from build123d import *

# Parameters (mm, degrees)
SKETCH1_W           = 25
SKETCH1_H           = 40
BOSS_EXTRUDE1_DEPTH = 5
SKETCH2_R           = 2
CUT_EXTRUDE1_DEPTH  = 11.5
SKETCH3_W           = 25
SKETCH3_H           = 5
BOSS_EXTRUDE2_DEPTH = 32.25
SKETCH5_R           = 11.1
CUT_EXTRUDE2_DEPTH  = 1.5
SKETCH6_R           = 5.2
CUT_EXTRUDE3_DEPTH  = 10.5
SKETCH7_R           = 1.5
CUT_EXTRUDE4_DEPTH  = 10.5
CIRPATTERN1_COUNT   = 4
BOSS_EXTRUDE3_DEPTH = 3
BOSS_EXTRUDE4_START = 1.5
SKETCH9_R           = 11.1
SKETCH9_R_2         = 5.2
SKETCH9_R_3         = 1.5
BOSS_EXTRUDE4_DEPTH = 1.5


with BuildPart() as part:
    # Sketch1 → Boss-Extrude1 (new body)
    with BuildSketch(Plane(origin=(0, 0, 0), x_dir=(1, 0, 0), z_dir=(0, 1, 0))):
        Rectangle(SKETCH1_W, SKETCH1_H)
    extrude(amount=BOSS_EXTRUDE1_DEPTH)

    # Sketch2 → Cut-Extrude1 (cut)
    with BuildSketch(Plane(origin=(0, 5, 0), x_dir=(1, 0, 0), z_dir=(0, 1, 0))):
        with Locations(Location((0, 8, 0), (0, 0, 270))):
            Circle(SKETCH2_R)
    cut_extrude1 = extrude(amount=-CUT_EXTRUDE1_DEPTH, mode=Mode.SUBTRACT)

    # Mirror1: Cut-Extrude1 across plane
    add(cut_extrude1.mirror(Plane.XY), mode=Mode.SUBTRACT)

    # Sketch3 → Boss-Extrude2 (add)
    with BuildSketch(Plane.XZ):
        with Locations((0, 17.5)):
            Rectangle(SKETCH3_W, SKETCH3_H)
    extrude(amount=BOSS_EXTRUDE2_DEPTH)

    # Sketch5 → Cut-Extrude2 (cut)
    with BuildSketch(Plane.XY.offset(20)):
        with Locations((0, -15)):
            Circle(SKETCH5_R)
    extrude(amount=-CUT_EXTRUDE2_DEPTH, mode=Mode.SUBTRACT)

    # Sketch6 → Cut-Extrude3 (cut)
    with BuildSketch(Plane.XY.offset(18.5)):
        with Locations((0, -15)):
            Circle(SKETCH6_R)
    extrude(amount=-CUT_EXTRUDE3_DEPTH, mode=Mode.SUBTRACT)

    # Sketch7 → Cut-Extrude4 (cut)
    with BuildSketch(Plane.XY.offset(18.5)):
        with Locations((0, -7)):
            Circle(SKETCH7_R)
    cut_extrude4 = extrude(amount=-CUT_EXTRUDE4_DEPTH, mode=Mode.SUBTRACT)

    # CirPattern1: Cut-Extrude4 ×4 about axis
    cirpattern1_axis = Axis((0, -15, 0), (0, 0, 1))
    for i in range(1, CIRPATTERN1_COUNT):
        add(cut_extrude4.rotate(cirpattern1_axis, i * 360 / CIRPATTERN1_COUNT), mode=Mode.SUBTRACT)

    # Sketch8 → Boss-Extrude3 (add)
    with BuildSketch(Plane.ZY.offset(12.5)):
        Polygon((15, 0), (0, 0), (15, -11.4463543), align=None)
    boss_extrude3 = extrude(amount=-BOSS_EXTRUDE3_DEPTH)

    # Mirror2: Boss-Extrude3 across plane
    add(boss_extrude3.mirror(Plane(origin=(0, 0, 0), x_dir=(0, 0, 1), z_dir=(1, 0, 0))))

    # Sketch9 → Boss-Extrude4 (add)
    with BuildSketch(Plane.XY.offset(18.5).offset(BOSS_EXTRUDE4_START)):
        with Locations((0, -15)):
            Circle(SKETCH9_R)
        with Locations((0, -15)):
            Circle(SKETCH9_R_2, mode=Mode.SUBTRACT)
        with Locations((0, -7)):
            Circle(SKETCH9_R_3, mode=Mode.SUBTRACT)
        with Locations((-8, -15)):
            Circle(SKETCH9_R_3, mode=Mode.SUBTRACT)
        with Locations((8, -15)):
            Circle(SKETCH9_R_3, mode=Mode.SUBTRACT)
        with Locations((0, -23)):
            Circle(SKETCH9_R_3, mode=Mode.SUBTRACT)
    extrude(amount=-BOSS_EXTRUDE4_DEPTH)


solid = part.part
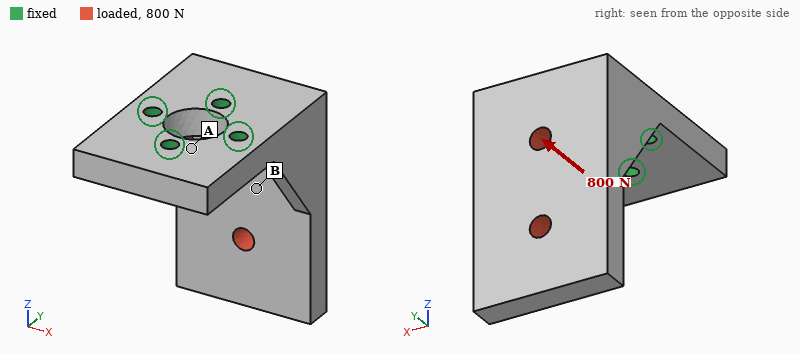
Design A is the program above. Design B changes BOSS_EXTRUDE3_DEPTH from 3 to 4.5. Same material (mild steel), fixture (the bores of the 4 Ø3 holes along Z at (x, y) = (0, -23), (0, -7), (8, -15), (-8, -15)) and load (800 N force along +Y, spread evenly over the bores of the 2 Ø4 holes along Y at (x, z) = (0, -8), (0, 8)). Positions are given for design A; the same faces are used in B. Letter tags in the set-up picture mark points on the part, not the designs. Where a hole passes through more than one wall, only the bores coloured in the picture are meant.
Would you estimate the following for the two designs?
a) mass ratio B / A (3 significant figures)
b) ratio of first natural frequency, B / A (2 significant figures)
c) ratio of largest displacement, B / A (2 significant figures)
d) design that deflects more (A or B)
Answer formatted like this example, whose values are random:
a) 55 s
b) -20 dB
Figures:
a) 1.03
b) 1.1
c) 0.85
d) A
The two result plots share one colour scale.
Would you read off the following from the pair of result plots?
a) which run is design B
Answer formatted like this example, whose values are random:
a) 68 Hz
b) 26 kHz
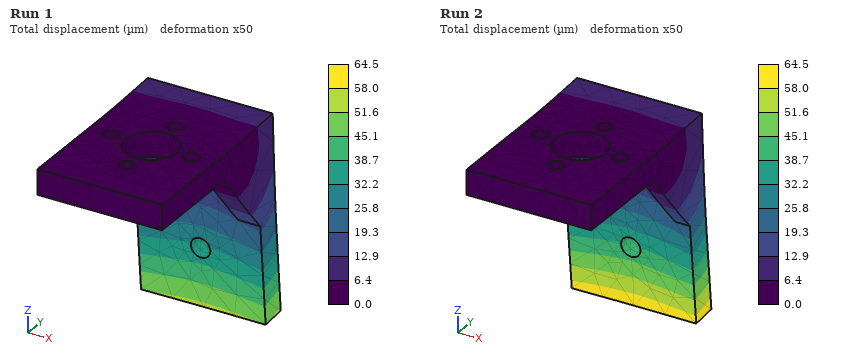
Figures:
a) Run 1
